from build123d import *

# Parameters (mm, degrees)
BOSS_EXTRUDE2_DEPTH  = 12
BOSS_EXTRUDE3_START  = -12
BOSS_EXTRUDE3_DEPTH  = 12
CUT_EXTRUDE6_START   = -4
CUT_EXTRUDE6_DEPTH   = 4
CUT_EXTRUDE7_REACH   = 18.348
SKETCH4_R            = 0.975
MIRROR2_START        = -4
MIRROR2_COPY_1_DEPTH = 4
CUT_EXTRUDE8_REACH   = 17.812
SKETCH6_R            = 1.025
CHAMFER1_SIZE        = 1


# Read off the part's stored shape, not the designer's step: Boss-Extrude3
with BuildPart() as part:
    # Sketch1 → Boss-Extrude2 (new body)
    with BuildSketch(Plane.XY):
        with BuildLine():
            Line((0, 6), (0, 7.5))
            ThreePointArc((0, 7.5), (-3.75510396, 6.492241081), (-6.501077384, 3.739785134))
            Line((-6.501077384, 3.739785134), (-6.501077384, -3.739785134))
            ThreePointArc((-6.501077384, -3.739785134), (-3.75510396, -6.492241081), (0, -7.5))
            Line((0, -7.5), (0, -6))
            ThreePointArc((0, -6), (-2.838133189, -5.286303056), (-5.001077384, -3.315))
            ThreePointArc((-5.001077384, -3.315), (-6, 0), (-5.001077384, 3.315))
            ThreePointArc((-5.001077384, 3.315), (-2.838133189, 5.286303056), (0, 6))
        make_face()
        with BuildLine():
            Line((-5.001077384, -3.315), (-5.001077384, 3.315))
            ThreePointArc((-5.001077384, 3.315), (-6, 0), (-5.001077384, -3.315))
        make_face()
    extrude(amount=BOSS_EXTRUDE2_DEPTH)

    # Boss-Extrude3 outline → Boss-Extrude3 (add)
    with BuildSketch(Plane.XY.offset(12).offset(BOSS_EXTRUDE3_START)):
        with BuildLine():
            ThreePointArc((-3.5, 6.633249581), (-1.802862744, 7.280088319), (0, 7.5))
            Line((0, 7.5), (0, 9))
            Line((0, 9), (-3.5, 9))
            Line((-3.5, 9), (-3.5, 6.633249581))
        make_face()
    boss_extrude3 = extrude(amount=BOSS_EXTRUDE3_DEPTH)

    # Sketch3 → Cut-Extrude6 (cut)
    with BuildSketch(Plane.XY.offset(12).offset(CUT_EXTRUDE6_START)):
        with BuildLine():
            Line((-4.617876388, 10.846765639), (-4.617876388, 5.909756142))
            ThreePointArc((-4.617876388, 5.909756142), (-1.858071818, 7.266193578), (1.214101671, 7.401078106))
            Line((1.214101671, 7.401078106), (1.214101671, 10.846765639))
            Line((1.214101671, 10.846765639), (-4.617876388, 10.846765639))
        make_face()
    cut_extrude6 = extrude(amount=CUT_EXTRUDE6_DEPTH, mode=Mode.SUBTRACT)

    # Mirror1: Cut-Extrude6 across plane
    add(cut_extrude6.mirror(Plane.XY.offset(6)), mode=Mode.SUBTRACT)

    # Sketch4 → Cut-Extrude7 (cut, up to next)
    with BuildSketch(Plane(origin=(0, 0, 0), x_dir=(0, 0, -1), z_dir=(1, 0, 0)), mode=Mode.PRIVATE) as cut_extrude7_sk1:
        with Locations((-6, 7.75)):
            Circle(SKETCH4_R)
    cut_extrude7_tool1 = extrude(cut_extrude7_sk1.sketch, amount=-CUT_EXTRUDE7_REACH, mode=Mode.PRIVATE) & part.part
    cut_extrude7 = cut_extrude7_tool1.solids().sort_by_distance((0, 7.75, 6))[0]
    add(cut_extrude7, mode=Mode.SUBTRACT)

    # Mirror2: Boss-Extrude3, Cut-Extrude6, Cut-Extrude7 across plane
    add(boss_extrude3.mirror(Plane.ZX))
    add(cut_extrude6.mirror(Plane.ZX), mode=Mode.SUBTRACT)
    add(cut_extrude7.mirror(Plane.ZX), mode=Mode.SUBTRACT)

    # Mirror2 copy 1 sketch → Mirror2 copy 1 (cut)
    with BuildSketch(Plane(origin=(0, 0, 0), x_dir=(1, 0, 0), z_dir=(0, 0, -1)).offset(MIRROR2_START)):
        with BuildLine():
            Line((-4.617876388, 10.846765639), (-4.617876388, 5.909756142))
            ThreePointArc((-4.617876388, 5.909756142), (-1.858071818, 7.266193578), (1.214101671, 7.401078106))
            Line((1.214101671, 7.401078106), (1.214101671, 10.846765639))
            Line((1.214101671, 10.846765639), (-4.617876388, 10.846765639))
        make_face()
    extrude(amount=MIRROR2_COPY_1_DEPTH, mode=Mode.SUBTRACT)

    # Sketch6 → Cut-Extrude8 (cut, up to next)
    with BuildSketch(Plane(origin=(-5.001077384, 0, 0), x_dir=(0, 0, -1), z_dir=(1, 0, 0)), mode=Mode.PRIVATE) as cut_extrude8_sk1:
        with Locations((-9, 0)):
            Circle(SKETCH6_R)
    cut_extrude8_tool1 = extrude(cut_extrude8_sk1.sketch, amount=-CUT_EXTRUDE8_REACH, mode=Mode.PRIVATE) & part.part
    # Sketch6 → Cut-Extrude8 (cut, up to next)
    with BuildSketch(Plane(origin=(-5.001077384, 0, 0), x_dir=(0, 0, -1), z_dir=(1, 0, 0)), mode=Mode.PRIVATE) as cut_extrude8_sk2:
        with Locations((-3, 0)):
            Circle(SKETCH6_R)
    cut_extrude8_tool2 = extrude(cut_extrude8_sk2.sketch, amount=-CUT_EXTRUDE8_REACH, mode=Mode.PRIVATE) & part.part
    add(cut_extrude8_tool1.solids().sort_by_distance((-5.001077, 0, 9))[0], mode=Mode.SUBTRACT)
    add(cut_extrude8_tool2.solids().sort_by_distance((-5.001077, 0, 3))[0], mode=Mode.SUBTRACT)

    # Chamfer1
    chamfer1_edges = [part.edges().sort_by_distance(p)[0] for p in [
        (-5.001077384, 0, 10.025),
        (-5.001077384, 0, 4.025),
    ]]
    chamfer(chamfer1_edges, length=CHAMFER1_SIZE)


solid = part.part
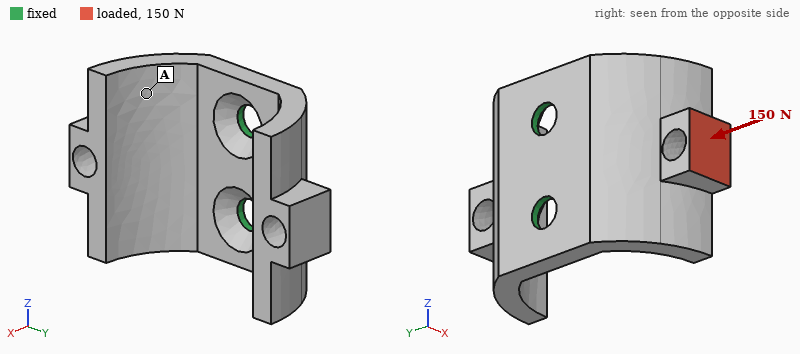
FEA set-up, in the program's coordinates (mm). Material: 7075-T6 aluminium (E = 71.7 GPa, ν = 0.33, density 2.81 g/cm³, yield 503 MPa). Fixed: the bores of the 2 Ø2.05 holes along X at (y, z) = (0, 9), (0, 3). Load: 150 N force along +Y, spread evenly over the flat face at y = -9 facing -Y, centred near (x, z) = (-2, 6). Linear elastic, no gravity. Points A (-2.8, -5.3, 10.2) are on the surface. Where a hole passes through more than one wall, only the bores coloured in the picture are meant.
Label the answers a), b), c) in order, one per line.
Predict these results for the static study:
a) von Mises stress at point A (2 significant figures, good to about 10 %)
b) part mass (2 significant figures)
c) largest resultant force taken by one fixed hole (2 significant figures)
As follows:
a) 51 MPa
b) 1.1 g
c) 77 N
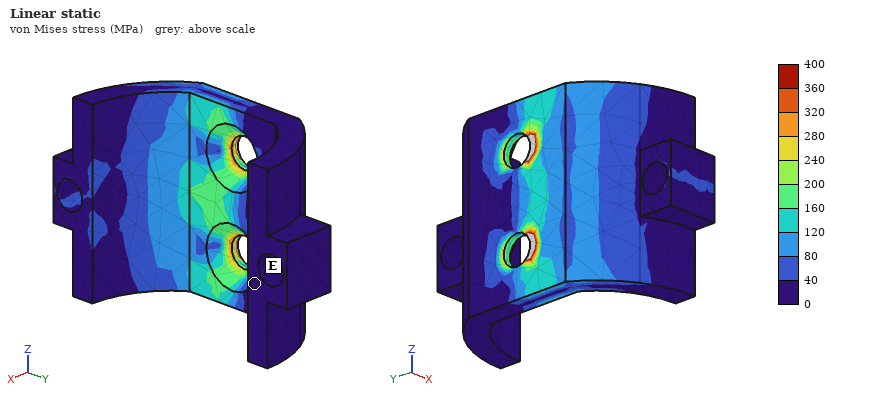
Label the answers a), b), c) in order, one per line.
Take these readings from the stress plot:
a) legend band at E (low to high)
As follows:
a) 0 to 40 MPa
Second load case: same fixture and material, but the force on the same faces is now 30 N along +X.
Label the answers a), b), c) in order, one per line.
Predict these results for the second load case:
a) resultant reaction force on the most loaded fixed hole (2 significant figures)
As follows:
a) 15 N
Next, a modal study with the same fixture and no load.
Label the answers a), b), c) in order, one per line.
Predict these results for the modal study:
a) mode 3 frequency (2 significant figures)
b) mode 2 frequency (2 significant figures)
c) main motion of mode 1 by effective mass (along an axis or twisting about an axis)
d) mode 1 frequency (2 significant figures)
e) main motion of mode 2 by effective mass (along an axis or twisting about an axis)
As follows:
a) 19 kHz
b) 10 kHz
c) along Y
d) 7500 Hz
e) along X
